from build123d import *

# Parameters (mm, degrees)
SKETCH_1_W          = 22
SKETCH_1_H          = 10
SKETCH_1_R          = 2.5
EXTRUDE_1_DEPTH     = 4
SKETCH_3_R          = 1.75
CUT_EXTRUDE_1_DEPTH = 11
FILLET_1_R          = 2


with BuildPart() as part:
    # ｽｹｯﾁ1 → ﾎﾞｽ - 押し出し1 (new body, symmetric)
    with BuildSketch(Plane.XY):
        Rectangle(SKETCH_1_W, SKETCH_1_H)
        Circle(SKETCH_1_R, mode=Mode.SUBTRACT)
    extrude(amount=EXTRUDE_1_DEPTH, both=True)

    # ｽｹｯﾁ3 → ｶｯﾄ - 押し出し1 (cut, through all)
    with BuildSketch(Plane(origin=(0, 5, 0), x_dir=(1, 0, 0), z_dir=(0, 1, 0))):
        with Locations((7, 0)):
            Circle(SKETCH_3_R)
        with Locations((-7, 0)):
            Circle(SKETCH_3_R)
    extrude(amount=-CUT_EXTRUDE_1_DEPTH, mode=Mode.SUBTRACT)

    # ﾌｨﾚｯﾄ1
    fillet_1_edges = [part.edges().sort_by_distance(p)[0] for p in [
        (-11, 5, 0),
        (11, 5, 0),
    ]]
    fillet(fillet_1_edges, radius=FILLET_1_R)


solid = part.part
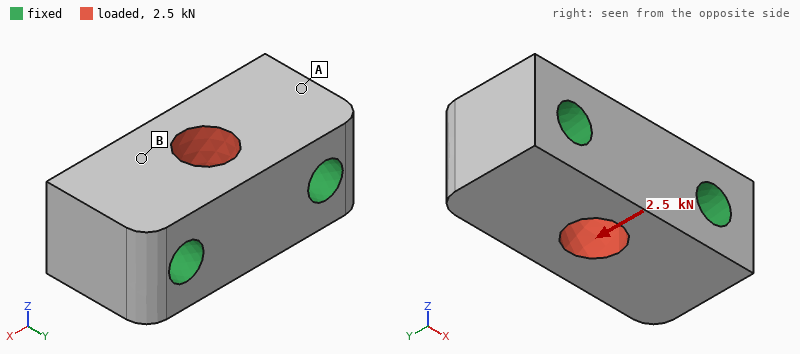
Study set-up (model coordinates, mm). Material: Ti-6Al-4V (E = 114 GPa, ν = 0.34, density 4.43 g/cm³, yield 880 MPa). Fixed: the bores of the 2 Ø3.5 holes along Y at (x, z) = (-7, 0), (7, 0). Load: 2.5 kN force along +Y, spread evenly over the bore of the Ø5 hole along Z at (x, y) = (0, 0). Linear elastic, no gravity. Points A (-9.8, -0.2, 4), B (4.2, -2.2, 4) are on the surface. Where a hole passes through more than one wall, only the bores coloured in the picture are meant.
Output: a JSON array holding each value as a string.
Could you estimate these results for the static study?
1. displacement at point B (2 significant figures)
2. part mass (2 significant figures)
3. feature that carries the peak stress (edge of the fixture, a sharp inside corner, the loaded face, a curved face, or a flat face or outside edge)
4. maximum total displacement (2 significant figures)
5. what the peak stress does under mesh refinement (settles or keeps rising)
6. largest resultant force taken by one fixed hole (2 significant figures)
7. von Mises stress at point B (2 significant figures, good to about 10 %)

["0.93 µm", "6.2 g", "edge of the fixture", "2.8 µm", "keeps rising", "1.3 kN", "23 MPa"]
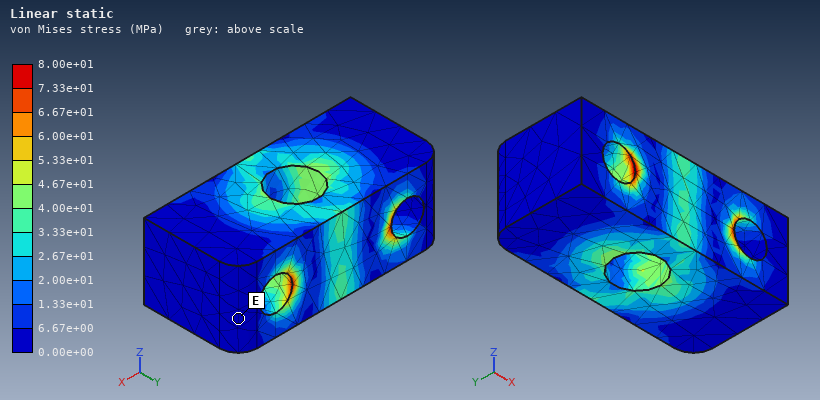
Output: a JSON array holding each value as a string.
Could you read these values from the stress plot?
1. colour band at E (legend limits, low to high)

["0.00e+00 to 6.67e+00 MPa"]
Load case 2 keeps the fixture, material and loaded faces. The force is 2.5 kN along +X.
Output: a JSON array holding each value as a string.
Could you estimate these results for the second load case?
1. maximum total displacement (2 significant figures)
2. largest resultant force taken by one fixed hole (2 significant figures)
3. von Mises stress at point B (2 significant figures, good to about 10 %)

["0.98 µm", "1.3 kN", "14 MPa"]
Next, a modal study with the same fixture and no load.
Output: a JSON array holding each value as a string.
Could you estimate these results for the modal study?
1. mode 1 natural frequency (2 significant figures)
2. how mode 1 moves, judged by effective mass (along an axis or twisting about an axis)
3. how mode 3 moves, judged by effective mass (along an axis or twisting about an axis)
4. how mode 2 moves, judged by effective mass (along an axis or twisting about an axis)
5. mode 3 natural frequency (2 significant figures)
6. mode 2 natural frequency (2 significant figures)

["110 kHz", "along Z", "along Y", "twisting about X", "130 kHz", "120 kHz"]
